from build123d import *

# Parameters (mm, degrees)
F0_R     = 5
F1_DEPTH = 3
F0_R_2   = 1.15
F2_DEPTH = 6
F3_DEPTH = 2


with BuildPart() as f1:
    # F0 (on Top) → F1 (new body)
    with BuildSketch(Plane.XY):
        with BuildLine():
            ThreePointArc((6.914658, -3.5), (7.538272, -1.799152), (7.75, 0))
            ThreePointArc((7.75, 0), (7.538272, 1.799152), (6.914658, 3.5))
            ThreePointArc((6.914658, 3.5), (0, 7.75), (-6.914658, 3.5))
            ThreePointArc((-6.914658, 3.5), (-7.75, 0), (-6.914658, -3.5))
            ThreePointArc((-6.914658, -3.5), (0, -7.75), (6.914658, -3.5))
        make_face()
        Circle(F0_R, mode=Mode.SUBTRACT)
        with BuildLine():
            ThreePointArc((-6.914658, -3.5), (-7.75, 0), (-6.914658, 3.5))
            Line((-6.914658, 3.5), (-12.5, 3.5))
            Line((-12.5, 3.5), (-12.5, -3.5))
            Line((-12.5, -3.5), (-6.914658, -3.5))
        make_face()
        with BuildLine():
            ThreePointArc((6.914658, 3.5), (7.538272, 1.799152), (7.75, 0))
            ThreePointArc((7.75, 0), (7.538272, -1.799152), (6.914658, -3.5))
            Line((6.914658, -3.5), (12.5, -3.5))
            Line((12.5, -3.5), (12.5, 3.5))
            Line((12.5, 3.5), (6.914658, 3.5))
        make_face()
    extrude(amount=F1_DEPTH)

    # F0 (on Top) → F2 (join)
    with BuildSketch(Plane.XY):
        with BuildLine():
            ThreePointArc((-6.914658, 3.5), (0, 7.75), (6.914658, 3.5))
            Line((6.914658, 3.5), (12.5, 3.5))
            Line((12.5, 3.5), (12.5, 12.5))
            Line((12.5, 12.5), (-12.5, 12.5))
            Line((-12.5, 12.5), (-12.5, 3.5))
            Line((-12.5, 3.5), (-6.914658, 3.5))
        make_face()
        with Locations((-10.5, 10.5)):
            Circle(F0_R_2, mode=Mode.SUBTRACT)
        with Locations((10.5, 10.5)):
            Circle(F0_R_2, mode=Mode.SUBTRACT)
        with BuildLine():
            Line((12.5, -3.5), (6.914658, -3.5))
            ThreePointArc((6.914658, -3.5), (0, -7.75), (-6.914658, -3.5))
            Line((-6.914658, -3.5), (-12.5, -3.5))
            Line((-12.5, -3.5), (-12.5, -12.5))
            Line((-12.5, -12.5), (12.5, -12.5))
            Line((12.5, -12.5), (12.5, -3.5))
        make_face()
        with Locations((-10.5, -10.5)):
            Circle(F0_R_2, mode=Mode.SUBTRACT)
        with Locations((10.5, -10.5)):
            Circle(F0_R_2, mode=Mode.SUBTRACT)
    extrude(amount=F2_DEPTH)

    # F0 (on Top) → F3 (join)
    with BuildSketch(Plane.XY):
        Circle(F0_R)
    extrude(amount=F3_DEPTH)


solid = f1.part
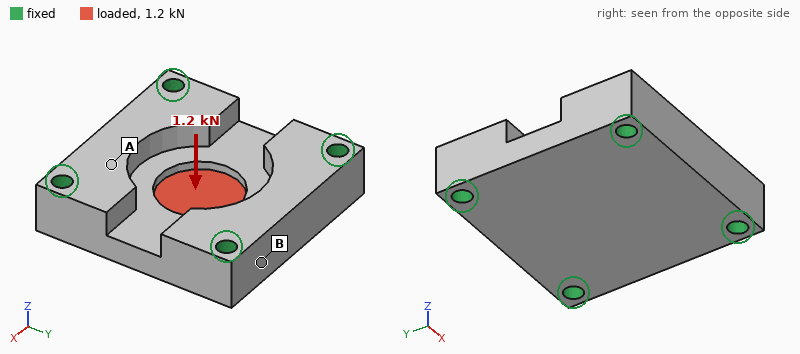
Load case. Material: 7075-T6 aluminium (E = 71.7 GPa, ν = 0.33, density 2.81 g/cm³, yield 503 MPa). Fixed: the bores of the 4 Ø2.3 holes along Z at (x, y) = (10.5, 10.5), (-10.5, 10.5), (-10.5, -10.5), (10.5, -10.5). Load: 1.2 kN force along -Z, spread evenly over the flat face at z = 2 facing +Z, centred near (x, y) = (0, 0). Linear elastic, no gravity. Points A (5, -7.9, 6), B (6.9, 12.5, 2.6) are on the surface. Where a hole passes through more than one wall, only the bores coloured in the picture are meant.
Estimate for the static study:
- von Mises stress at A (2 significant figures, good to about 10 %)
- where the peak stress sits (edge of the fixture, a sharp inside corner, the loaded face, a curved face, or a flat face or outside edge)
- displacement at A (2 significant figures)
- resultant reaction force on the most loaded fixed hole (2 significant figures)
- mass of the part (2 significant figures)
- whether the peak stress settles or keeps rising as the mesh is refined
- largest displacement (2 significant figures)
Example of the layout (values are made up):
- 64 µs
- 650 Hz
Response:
- 21 MPa
- edge of the fixture
- 4.9 µm
- 440 N
- 7.9 g
- keeps rising
- 22 µm
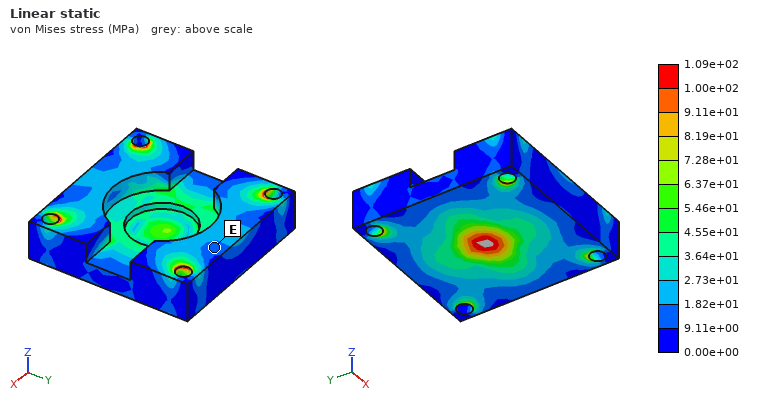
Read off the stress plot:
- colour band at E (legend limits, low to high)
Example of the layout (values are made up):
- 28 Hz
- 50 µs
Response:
- 9.11e+00 to 1.82e+01 MPa
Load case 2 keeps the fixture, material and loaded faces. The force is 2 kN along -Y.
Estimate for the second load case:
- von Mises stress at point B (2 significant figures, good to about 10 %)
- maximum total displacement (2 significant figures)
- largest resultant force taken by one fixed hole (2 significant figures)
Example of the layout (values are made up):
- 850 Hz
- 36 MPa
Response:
- 7.8 MPa
- 8.3 µm
- 560 N
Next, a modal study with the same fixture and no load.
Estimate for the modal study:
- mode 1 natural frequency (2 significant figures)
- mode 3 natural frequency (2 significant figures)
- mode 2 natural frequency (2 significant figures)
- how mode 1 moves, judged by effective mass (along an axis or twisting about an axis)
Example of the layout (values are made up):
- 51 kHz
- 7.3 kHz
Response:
- 38 kHz
- 54 kHz
- 49 kHz
- along Z
